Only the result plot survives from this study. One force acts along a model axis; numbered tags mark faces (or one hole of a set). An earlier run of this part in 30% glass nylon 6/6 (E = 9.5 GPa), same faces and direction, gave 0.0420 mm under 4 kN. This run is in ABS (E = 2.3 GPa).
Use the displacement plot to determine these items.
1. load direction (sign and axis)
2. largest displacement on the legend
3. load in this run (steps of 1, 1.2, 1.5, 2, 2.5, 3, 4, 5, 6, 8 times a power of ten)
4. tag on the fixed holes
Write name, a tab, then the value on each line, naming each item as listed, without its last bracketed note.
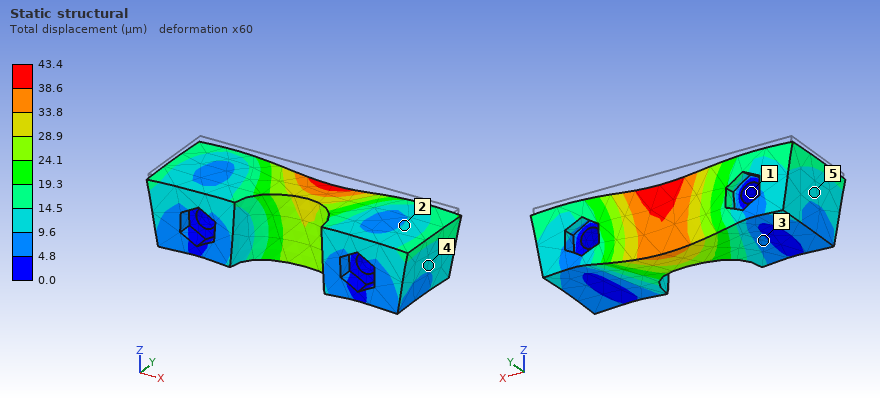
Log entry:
load direction	-Z
largest displacement on the legend	43.4 µm
load in this run	1 kN
tag on the fixed holes	1
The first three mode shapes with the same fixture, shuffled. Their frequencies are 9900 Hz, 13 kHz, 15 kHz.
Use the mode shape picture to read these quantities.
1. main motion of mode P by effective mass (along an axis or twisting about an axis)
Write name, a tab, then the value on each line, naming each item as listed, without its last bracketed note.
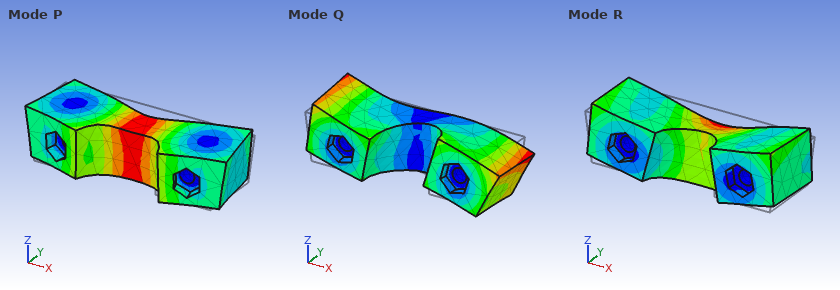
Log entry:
main motion of mode P by effective mass	along Y
